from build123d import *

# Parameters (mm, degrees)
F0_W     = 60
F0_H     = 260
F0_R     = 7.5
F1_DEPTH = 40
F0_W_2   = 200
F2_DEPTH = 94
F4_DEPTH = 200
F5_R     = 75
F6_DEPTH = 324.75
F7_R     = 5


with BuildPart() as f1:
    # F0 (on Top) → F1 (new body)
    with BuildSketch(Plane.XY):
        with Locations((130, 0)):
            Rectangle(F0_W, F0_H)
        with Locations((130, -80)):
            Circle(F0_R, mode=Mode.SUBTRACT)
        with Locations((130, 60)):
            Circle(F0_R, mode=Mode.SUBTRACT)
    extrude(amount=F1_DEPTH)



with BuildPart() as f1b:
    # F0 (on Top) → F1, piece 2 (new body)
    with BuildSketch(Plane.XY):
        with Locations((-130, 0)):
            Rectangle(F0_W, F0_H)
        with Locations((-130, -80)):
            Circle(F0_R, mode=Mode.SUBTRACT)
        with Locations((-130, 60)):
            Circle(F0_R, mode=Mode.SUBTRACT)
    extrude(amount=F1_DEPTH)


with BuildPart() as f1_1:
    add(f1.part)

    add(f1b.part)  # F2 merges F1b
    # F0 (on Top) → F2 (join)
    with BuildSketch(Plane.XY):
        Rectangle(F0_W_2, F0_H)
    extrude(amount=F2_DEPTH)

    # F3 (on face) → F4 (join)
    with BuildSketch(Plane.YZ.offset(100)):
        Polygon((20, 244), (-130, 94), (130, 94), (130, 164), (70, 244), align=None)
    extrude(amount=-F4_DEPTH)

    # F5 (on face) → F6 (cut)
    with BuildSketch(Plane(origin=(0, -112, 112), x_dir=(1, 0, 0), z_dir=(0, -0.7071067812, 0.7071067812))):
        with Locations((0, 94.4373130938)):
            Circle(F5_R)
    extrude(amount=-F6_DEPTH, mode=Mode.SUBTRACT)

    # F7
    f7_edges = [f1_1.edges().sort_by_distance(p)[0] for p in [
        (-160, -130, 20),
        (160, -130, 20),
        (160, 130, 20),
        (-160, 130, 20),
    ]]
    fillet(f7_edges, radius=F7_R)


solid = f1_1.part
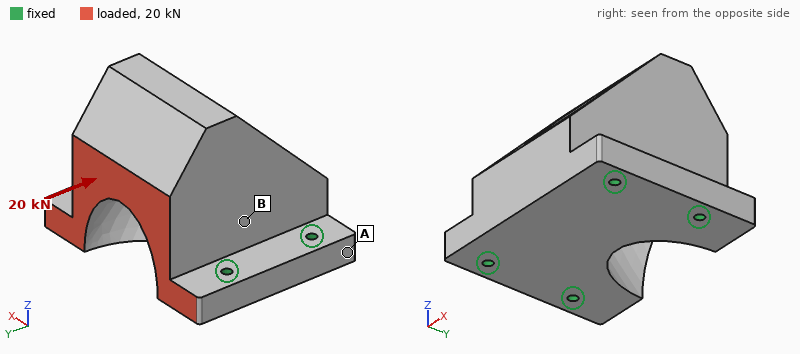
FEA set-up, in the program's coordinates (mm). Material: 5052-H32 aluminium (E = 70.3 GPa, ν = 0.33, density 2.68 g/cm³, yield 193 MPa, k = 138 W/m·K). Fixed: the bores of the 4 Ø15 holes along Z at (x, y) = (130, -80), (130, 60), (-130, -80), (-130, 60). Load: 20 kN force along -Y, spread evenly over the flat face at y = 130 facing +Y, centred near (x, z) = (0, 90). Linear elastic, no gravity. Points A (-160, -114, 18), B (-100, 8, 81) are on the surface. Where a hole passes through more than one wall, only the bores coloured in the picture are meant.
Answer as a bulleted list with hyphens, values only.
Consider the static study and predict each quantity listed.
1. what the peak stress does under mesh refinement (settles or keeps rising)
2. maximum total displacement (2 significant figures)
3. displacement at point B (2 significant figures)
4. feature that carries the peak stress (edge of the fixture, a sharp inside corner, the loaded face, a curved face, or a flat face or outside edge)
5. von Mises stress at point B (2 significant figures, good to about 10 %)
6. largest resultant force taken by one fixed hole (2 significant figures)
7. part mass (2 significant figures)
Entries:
- keeps rising
- 26 µm
- 8.8 µm
- edge of the fixture
- 2.2 MPa
- 7.5 kN
- 20 kg
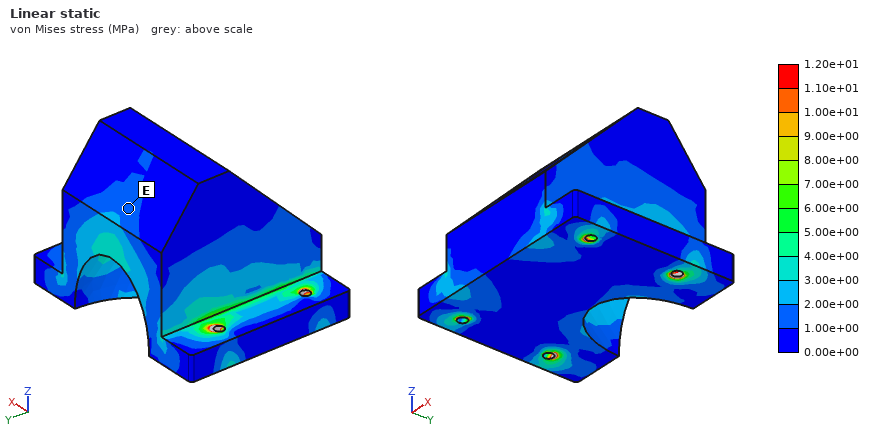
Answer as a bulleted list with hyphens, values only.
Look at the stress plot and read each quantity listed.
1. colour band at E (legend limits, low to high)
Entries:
- 1.00e+00 to 2.00e+00 MPa
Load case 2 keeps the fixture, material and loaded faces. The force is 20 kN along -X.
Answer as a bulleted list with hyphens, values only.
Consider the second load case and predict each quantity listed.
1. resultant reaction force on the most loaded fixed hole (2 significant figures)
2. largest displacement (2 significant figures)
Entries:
- 11 kN
- 42 µm
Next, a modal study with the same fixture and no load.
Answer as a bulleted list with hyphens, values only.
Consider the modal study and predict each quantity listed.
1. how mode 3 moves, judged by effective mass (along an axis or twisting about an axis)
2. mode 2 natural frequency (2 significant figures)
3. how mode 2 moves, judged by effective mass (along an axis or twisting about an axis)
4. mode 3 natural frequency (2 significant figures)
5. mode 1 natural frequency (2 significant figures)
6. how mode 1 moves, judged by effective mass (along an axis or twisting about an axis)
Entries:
- along Z
- 1400 Hz
- along X
- 2200 Hz
- 1200 Hz
- along Y
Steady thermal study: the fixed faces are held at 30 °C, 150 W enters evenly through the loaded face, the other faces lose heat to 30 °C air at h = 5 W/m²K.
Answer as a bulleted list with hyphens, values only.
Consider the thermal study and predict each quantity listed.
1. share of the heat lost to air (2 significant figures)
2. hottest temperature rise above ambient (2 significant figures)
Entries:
- 5.8 %
- 13 K
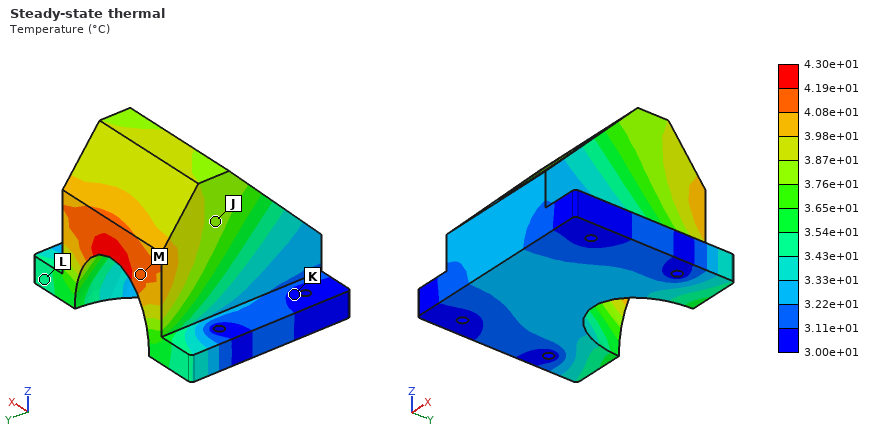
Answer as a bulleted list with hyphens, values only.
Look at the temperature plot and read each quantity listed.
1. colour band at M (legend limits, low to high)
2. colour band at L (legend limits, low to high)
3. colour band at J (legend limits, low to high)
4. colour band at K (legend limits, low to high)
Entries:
- 4.08e+01 to 4.19e+01 °C
- 3.43e+01 to 3.54e+01 °C
- 3.76e+01 to 3.87e+01 °C
- 3.00e+01 to 3.11e+01 °C
